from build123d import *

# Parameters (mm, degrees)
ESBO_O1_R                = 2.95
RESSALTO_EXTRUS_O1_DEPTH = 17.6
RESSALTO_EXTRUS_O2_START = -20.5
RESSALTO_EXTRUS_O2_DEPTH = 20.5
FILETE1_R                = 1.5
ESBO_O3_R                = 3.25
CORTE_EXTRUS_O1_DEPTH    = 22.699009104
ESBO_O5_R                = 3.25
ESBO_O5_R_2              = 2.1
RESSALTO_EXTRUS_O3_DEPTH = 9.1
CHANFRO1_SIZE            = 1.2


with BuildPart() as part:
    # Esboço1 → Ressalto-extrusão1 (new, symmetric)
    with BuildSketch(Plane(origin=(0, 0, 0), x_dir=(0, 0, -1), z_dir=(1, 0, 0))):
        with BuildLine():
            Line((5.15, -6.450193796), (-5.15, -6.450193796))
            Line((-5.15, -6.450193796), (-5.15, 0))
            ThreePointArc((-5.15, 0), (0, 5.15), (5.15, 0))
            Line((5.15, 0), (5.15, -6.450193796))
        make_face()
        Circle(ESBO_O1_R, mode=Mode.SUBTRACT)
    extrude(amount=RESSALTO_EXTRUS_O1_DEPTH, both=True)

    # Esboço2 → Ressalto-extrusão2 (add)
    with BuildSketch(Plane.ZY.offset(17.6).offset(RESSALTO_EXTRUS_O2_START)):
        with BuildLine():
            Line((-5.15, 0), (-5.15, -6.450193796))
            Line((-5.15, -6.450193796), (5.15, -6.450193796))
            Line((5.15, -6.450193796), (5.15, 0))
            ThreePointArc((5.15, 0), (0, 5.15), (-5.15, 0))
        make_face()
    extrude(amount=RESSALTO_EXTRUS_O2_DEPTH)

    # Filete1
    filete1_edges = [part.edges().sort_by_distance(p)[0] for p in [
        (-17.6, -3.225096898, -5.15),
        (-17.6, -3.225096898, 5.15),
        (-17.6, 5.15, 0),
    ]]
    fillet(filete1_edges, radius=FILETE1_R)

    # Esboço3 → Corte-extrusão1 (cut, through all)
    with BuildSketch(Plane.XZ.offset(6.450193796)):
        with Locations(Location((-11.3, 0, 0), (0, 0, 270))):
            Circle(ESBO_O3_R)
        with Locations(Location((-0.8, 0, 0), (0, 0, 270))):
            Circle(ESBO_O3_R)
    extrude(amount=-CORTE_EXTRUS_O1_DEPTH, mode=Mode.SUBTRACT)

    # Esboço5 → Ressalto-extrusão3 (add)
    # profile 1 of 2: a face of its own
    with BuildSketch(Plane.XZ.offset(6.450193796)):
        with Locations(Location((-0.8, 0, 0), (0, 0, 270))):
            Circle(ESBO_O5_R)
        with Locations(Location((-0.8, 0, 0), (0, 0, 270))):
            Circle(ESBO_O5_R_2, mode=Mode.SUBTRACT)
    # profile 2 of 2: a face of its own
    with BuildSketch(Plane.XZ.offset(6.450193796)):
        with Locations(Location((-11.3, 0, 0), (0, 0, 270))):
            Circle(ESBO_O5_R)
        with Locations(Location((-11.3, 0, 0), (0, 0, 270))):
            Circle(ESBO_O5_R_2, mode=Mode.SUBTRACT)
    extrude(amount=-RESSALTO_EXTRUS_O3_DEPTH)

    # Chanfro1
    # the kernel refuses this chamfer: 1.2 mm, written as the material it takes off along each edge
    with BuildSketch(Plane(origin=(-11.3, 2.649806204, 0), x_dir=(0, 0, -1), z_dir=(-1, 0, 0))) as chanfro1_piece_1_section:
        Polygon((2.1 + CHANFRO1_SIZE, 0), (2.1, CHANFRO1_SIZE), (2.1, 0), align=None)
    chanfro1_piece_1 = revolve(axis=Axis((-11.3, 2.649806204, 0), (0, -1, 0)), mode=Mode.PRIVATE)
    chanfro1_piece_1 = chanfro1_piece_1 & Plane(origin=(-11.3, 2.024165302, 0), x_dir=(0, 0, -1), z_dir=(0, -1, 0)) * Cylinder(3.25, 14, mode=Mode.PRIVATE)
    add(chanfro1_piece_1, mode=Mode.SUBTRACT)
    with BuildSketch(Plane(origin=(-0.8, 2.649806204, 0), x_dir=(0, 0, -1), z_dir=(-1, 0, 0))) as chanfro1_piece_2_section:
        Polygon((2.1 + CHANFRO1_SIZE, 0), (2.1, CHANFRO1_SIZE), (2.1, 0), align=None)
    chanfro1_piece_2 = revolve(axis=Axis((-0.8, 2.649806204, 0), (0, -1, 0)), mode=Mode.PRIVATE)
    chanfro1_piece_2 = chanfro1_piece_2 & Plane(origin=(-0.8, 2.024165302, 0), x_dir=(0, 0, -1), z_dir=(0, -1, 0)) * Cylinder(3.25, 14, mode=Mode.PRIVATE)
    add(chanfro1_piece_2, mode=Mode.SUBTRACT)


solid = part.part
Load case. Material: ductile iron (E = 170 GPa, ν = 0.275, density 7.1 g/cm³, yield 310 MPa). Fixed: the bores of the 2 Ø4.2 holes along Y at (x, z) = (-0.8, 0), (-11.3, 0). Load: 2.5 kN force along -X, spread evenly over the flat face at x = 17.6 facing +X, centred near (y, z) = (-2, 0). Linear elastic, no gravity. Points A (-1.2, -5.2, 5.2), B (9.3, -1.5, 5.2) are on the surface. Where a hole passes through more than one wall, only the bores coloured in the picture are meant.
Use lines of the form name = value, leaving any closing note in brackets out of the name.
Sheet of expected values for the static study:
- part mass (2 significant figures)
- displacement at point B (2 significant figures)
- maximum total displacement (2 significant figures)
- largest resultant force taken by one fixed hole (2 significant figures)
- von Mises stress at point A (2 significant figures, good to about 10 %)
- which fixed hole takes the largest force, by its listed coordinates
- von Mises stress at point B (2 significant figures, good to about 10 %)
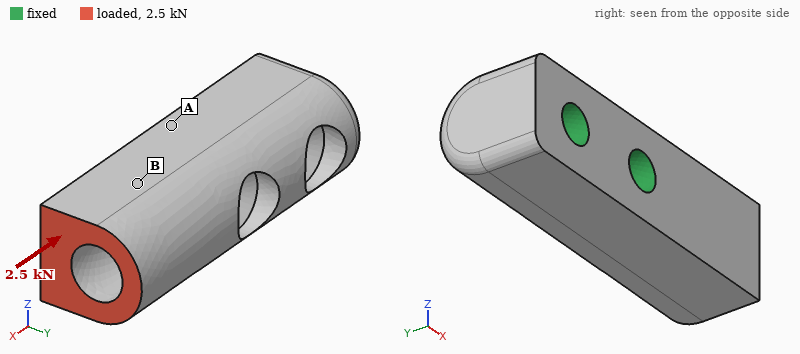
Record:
part mass = 21 g
displacement at point B = 2.5 µm
maximum total displacement = 5.7 µm
largest resultant force taken by one fixed hole = 2.2 kN
von Mises stress at point A = 13 MPa
which fixed hole takes the largest force, by its listed coordinates = (-0.8, 0)
von Mises stress at point B = 34 MPa
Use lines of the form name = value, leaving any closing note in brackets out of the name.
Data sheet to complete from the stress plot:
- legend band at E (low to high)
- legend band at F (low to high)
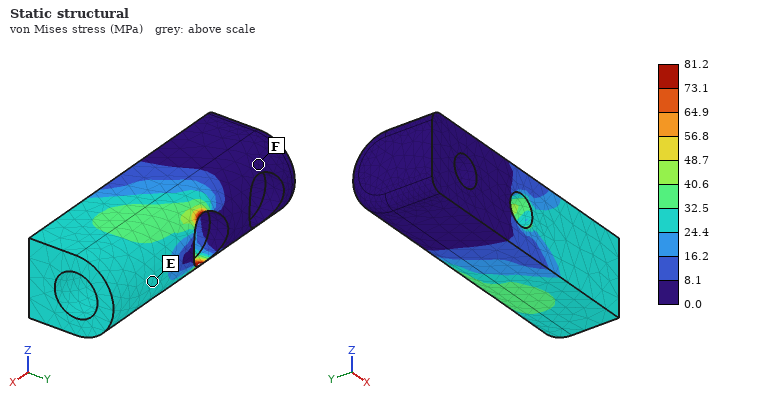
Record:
legend band at E = 24.4 to 32.5 MPa
legend band at F = 0.0 to 8.1 MPa
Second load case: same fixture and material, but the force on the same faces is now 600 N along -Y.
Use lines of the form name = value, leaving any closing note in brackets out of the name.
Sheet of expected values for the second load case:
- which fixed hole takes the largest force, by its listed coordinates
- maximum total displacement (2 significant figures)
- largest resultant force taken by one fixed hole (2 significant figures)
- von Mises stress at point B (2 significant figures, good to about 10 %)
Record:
which fixed hole takes the largest force, by its listed coordinates = (-0.8, 0)
maximum total displacement = 16 µm
largest resultant force taken by one fixed hole = 790 N
von Mises stress at point B = 28 MPa
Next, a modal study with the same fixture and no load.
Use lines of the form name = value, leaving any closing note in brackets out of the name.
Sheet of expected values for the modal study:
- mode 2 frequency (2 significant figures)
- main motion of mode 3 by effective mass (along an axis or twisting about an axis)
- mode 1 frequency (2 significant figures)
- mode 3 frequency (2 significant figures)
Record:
mode 2 frequency = 18 kHz
main motion of mode 3 by effective mass = twisting about X
mode 1 frequency = 18 kHz
mode 3 frequency = 37 kHz
